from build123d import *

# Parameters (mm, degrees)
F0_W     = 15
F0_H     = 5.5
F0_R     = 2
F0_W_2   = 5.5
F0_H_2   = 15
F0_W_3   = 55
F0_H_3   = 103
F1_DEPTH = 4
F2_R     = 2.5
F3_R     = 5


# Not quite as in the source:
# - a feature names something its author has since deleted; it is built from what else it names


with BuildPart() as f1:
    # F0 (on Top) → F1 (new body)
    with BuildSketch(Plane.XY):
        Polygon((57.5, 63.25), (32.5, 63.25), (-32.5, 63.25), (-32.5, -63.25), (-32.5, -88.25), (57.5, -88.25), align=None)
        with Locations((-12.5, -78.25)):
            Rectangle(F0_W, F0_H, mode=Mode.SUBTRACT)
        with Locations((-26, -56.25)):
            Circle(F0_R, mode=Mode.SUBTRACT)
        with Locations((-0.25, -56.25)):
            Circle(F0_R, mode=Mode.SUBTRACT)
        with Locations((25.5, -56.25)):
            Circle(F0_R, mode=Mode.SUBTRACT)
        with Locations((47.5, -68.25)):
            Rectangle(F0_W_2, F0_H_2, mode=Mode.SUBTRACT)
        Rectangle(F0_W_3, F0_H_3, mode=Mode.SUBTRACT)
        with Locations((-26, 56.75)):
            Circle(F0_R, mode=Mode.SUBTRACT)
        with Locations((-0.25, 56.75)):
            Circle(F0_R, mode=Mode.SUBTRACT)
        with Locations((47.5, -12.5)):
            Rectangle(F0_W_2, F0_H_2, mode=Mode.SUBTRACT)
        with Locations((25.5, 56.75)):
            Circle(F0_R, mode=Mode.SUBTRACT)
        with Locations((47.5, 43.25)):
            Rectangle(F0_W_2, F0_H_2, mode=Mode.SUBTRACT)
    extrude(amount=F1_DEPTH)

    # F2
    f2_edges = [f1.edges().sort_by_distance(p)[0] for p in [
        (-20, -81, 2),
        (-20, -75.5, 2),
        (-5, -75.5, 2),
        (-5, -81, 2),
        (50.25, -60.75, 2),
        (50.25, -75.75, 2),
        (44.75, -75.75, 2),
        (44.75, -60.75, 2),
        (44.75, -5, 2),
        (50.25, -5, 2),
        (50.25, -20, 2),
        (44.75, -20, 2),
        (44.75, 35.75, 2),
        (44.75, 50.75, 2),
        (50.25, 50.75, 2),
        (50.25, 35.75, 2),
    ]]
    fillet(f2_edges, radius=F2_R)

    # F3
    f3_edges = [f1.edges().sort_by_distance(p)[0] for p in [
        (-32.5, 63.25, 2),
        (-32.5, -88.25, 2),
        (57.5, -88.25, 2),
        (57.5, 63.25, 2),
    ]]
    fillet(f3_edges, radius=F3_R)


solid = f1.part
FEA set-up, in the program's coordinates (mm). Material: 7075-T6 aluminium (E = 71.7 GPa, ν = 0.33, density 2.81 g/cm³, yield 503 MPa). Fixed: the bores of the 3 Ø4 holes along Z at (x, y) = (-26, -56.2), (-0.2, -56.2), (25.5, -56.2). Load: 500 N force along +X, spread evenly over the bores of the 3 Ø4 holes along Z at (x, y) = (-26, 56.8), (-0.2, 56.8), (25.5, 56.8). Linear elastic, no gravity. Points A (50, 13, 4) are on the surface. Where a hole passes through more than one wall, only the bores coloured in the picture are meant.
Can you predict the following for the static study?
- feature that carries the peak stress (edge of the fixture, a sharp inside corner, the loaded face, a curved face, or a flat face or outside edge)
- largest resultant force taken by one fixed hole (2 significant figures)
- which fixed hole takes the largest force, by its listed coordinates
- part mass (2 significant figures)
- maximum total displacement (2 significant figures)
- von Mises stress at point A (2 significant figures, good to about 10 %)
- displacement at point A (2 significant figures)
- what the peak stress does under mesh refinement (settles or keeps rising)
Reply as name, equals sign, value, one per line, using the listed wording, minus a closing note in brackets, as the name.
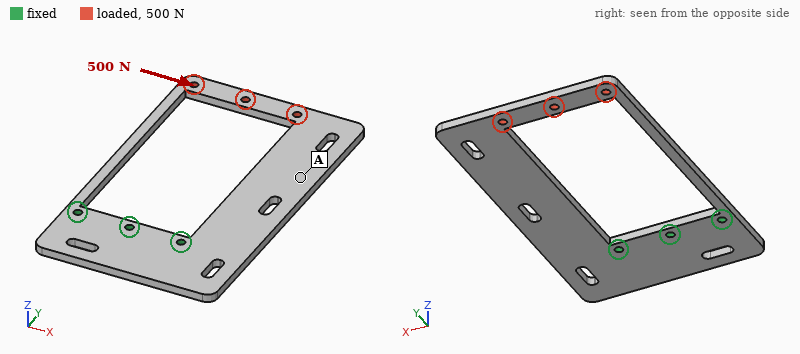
feature that carries the peak stress = a sharp inside corner
largest resultant force taken by one fixed hole = 2.0 kN
which fixed hole takes the largest force, by its listed coordinates = (25.5, -56.2)
part mass = 85 g
maximum total displacement = 0.58 mm
von Mises stress at point A = 14 MPa
displacement at point A = 0.31 mm
what the peak stress does under mesh refinement = keeps rising
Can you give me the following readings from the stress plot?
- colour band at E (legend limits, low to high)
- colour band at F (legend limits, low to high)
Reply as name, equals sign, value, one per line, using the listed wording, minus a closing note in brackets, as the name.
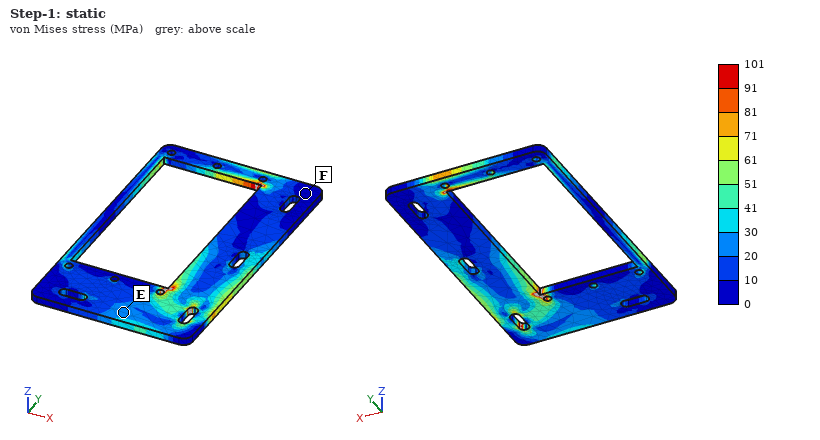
colour band at E = 20 to 30 MPa
colour band at F = 0 to 10 MPa
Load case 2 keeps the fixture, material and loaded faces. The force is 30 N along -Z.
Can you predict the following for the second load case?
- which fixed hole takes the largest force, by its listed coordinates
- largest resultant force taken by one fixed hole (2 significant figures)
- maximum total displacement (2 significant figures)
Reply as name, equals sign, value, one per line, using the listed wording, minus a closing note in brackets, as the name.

which fixed hole takes the largest force, by its listed coordinates = (-26, -56.2)
largest resultant force taken by one fixed hole = 14 N
maximum total displacement = 1.7 mm
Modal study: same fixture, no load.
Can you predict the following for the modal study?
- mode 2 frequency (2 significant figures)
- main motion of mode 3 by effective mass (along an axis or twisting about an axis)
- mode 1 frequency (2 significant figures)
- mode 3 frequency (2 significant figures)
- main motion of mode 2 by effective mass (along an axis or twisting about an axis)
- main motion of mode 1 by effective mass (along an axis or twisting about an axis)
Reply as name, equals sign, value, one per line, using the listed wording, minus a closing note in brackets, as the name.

mode 2 frequency = 450 Hz
main motion of mode 3 by effective mass = along X
mode 1 frequency = 170 Hz
mode 3 frequency = 990 Hz
main motion of mode 2 by effective mass = twisting about Y
main motion of mode 1 by effective mass = along Z
